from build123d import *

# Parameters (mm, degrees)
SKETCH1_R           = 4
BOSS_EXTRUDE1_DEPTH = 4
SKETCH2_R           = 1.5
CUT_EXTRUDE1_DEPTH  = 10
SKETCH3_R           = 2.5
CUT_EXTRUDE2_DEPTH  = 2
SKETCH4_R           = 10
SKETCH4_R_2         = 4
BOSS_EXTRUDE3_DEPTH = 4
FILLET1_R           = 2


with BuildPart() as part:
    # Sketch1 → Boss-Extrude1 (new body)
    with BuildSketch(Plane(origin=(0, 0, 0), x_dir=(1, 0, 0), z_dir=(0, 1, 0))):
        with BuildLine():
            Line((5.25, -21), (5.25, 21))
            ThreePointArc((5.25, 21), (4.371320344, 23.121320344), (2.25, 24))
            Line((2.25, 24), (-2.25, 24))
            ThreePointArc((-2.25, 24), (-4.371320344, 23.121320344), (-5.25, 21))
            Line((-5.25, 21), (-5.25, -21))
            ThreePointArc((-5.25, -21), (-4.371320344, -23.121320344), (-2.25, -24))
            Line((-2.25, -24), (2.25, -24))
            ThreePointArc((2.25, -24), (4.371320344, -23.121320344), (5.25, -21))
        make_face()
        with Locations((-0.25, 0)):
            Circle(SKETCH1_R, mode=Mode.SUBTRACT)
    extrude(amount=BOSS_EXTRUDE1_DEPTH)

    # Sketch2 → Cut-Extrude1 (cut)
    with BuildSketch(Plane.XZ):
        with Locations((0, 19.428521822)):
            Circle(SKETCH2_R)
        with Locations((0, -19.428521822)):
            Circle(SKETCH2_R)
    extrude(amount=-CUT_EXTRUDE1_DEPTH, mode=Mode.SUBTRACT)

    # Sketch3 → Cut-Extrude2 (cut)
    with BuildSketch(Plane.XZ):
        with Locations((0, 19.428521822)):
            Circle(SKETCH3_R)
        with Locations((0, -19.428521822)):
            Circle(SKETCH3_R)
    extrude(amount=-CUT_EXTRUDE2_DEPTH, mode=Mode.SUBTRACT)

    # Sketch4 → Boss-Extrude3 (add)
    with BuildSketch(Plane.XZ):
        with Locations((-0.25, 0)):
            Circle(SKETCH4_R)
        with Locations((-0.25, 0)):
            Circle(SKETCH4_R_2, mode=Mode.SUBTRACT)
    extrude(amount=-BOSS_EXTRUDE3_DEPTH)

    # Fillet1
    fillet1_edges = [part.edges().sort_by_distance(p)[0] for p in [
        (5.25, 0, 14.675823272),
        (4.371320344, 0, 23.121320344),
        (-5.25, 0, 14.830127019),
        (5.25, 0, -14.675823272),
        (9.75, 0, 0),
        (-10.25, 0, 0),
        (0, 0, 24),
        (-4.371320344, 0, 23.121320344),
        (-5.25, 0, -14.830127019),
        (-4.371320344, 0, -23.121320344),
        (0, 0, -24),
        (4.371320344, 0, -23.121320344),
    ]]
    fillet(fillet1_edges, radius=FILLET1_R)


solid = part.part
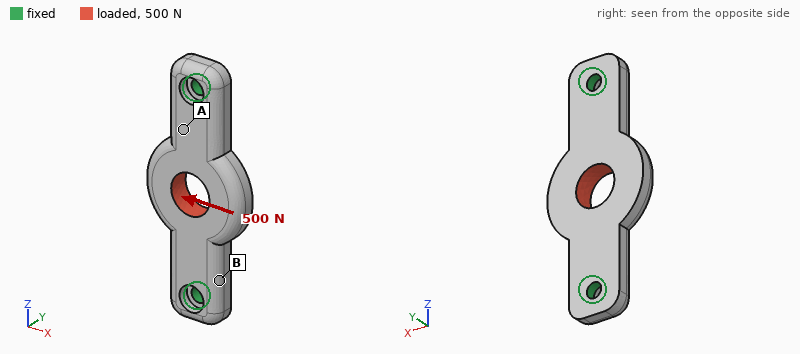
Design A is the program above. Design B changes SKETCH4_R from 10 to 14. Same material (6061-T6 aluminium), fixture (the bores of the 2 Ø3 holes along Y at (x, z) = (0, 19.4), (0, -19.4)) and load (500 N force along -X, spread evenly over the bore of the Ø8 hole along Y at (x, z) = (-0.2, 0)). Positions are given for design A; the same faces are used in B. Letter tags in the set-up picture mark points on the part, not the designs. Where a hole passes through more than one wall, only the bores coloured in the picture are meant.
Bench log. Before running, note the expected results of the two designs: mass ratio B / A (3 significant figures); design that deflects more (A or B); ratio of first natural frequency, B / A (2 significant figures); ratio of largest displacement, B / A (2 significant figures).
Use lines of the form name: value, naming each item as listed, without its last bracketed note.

mass ratio B / A: 1.42
design that deflects more: A
ratio of first natural frequency, B / A: 0.76
ratio of largest displacement, B / A: 0.76
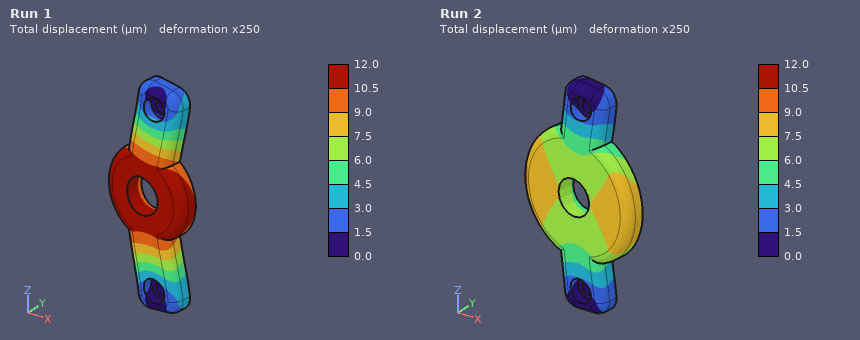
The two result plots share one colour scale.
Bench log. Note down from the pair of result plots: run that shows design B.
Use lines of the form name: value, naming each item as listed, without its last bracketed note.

run that shows design B: Run 2
